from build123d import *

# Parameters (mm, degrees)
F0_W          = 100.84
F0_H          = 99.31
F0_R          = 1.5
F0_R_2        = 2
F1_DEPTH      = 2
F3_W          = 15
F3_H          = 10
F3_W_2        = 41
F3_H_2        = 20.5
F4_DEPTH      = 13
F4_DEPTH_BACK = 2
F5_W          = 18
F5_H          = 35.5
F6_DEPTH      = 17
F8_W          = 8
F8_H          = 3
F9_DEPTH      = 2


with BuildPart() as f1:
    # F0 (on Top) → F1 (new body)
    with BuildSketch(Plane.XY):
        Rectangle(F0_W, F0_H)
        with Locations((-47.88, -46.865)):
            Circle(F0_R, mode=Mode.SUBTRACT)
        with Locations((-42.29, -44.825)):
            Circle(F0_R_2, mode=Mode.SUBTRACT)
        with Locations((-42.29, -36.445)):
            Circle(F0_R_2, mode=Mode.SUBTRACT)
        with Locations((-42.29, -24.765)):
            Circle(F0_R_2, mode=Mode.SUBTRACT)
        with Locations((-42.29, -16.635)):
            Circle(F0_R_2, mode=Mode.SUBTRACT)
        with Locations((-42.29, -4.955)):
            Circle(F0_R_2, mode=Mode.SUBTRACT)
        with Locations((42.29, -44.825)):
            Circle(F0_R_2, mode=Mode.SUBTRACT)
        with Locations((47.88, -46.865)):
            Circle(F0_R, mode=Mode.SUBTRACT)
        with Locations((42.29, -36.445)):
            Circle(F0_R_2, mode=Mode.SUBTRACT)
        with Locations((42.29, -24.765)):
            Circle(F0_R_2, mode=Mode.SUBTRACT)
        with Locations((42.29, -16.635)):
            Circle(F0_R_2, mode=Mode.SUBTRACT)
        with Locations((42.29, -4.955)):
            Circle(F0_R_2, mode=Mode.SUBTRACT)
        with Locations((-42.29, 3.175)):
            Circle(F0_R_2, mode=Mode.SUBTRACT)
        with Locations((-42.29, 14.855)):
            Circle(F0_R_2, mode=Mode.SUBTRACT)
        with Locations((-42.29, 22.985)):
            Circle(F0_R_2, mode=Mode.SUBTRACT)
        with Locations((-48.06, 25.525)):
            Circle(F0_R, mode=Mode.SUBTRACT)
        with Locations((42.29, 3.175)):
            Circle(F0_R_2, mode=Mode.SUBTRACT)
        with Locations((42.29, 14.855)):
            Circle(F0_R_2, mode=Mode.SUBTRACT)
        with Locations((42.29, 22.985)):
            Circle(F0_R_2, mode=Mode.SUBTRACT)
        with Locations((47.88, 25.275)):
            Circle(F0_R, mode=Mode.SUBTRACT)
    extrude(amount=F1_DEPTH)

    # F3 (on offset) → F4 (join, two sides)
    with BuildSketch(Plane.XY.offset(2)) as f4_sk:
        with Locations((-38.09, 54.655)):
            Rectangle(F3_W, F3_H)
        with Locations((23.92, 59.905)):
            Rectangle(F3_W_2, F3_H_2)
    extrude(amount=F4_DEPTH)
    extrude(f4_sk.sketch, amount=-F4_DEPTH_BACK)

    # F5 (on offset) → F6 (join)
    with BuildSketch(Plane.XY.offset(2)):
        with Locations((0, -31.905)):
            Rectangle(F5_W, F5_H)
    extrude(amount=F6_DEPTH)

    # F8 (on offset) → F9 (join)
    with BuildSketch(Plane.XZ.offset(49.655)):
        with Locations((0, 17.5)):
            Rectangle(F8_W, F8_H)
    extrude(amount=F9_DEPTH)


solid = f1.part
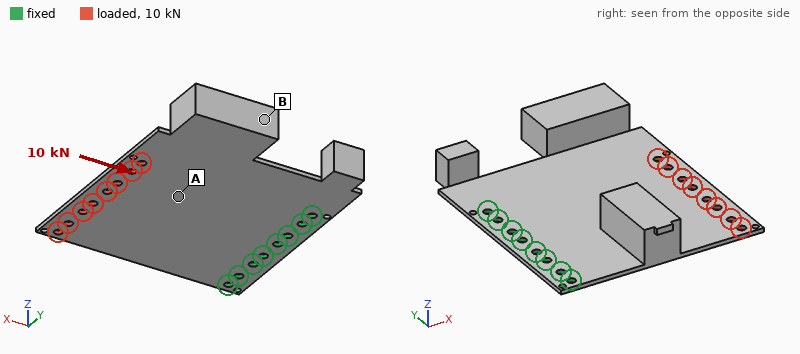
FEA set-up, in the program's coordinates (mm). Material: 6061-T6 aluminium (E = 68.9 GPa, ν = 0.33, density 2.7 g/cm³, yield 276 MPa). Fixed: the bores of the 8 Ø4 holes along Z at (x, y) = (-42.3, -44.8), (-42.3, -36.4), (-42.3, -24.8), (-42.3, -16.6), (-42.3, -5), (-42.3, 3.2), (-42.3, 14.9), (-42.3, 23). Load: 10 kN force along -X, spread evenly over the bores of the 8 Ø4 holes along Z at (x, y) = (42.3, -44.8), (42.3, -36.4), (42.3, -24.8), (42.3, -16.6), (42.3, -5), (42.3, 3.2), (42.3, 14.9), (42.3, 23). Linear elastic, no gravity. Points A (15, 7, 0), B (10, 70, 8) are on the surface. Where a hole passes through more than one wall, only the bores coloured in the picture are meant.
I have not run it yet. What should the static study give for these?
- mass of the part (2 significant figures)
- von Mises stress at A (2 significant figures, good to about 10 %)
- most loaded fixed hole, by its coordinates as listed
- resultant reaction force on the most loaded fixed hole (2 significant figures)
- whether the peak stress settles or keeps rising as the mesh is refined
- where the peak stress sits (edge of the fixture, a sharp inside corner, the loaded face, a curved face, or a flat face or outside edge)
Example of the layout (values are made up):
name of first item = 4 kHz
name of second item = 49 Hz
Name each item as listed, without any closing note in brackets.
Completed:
mass of the part = 120 g
von Mises stress at A = 60 MPa
most loaded fixed hole, by its coordinates as listed = (-42.3, 23)
resultant reaction force on the most loaded fixed hole = 1.8 kN
whether the peak stress settles or keeps rising as the mesh is refined = keeps rising
where the peak stress sits = edge of the fixture
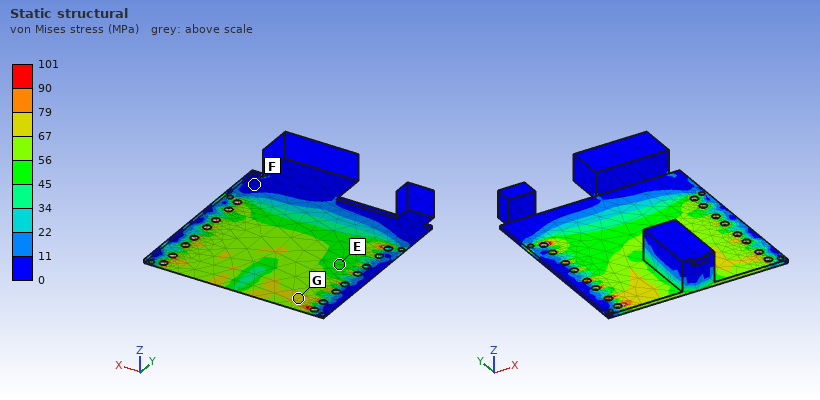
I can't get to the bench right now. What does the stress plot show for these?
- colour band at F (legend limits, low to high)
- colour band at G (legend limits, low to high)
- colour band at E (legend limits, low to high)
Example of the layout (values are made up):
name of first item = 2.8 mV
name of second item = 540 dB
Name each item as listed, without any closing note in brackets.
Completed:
colour band at F = 0 to 11 MPa
colour band at G = 67 to 79 MPa
colour band at E = 45 to 56 MPa
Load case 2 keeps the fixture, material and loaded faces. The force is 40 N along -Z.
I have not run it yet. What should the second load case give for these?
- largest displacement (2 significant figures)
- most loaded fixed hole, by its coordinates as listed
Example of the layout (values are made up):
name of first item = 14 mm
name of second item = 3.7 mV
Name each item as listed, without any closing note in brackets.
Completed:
largest displacement = 1.7 mm
most loaded fixed hole, by its coordinates as listed = (-42.3, 14.9)
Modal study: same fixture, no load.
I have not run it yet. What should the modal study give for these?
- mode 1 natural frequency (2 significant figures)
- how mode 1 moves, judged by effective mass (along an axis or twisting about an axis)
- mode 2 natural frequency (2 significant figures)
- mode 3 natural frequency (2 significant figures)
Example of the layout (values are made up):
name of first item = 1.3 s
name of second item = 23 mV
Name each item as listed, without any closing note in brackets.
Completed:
mode 1 natural frequency = 120 Hz
how mode 1 moves, judged by effective mass = along Z
mode 2 natural frequency = 240 Hz
mode 3 natural frequency = 600 Hz
